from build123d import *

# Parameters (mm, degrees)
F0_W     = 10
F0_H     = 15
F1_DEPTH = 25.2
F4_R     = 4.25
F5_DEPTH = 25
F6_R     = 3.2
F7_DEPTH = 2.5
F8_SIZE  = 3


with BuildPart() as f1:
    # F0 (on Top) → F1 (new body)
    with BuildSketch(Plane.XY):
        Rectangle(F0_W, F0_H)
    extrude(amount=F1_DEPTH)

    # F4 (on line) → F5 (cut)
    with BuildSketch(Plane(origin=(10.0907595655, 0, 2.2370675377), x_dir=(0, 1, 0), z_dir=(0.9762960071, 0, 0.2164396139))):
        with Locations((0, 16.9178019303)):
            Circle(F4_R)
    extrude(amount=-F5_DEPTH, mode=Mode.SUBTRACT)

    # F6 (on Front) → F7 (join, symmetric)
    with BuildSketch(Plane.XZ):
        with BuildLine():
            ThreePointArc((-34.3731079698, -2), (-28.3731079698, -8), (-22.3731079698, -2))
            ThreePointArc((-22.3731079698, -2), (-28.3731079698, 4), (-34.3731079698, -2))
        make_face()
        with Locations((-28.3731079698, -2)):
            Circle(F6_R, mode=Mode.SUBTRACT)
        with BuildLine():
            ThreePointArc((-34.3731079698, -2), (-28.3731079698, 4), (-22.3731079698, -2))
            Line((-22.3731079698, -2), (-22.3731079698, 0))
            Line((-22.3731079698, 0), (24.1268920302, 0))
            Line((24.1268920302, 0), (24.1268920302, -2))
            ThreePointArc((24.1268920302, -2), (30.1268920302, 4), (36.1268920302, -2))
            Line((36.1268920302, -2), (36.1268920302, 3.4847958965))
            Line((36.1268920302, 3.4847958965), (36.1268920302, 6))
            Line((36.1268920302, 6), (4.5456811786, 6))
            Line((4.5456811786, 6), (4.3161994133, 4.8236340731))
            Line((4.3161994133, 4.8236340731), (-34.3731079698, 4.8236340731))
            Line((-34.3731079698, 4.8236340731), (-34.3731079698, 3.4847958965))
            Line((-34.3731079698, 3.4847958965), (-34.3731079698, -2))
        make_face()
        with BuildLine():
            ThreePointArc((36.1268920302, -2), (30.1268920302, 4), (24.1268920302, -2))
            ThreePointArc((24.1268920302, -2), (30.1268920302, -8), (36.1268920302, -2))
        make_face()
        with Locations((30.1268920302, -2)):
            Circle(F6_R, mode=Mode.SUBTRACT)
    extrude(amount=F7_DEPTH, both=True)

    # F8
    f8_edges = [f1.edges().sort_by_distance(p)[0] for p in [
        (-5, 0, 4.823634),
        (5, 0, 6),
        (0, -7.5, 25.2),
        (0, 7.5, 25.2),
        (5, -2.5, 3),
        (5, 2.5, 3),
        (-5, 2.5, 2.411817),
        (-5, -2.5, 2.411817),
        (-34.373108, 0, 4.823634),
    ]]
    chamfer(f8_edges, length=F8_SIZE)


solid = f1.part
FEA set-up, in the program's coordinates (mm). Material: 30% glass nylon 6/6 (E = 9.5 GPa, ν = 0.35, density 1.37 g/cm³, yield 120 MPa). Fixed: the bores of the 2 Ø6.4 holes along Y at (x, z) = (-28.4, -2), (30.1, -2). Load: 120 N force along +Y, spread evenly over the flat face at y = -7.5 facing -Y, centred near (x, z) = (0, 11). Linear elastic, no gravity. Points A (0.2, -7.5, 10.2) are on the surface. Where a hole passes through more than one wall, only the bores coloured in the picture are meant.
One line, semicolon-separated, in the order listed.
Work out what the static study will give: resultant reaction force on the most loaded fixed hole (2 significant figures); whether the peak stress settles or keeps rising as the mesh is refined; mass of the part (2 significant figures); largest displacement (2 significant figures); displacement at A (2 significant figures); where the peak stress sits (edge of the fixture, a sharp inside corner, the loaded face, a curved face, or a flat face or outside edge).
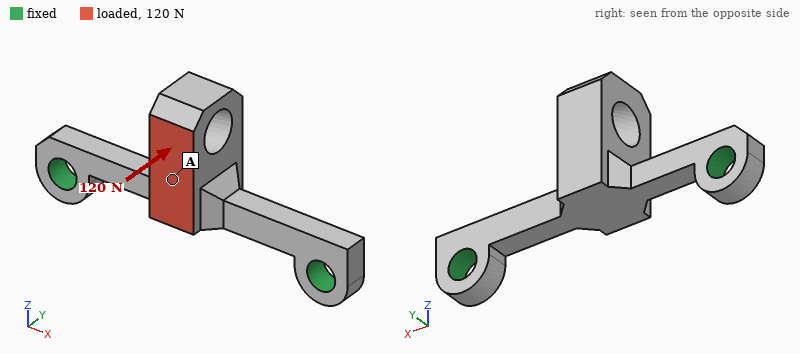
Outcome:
62 N; keeps rising; 7.4 g; 0.75 mm; 0.38 mm; a sharp inside corner
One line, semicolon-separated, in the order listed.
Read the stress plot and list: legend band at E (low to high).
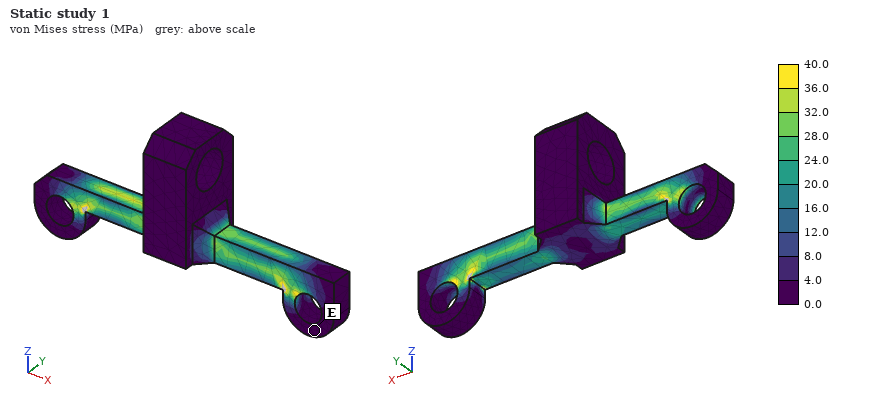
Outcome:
0.0 to 4.0 MPa
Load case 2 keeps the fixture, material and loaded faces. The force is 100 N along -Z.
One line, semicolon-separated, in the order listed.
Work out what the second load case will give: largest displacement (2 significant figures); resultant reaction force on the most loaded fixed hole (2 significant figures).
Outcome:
0.49 mm; 67 N
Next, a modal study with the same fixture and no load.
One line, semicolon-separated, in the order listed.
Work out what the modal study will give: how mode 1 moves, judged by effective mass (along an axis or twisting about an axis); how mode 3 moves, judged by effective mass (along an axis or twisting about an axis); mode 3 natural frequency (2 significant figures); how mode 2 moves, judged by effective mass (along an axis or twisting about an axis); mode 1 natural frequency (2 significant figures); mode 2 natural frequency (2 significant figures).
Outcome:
along Y; along Y; 3400 Hz; along Z; 1100 Hz; 2700 Hz
